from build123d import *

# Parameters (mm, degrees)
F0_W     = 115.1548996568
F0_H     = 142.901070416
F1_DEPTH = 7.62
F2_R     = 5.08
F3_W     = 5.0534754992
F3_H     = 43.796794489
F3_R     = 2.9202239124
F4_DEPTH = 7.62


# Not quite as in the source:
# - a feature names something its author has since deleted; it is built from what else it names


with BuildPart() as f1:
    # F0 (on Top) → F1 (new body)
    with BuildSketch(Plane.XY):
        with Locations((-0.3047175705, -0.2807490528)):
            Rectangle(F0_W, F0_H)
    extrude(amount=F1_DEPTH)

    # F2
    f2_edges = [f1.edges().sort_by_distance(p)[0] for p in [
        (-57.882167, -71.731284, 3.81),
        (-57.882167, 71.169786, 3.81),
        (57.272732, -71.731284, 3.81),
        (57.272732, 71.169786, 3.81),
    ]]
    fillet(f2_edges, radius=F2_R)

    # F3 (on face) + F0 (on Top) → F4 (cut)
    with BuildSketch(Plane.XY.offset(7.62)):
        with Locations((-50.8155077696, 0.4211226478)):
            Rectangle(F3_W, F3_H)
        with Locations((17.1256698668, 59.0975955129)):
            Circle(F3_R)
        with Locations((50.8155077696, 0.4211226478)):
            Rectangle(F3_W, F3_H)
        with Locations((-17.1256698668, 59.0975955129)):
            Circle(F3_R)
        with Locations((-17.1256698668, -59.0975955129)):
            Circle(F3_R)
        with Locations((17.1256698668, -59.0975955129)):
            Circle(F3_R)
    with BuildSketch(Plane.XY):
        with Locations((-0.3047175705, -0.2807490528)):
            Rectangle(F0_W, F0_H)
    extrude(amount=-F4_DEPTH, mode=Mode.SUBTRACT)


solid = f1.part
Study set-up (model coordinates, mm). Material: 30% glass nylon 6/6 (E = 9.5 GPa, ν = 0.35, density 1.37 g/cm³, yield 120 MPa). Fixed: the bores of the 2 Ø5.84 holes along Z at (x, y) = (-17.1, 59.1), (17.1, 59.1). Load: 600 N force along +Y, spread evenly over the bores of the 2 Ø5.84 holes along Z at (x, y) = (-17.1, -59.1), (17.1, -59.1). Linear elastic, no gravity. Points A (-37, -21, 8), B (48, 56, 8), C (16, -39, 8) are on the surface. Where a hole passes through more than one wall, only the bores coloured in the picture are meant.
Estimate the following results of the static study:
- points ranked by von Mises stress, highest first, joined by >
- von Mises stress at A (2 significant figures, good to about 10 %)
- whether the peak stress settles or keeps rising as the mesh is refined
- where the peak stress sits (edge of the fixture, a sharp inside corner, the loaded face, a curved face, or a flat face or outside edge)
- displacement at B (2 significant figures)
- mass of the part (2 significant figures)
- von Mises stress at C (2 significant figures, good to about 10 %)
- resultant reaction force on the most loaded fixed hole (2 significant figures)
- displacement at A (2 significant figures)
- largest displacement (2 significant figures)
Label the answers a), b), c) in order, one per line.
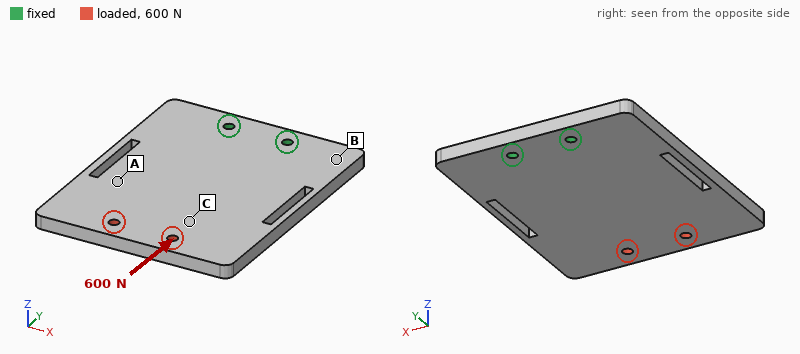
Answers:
a) C > A > B
b) 0.68 MPa
c) keeps rising
d) edge of the fixture
e) 5.6 µm
f) 170 g
g) 1.2 MPa
h) 300 N
i) 8.9 µm
j) 16 µm
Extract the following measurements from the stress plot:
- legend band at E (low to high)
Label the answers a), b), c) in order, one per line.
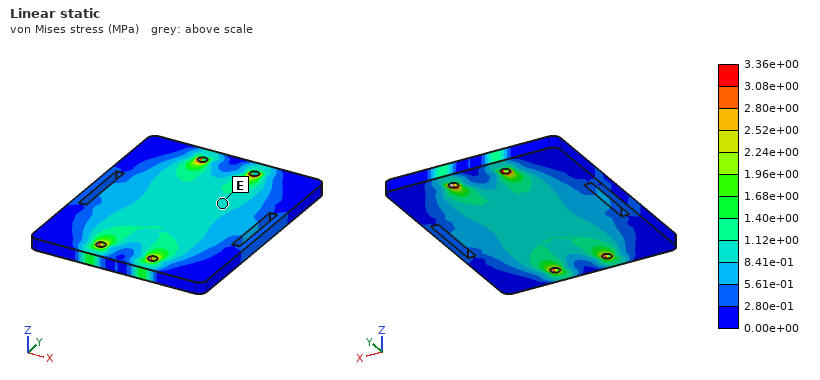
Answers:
a) 8.41e-01 to 1.12e+00 MPa
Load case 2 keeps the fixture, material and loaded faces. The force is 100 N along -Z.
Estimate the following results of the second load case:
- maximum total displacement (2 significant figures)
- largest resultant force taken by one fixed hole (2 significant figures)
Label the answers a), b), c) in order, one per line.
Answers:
a) 1.9 mm
b) 50 N
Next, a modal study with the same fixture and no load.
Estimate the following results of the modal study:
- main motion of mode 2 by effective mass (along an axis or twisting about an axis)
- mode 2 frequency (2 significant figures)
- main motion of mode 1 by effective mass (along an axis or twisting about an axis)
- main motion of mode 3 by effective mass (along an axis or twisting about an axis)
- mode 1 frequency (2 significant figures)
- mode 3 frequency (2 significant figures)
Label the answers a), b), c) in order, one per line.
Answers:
a) twisting about Y
b) 430 Hz
c) along Z
d) along X
e) 180 Hz
f) 960 Hz
